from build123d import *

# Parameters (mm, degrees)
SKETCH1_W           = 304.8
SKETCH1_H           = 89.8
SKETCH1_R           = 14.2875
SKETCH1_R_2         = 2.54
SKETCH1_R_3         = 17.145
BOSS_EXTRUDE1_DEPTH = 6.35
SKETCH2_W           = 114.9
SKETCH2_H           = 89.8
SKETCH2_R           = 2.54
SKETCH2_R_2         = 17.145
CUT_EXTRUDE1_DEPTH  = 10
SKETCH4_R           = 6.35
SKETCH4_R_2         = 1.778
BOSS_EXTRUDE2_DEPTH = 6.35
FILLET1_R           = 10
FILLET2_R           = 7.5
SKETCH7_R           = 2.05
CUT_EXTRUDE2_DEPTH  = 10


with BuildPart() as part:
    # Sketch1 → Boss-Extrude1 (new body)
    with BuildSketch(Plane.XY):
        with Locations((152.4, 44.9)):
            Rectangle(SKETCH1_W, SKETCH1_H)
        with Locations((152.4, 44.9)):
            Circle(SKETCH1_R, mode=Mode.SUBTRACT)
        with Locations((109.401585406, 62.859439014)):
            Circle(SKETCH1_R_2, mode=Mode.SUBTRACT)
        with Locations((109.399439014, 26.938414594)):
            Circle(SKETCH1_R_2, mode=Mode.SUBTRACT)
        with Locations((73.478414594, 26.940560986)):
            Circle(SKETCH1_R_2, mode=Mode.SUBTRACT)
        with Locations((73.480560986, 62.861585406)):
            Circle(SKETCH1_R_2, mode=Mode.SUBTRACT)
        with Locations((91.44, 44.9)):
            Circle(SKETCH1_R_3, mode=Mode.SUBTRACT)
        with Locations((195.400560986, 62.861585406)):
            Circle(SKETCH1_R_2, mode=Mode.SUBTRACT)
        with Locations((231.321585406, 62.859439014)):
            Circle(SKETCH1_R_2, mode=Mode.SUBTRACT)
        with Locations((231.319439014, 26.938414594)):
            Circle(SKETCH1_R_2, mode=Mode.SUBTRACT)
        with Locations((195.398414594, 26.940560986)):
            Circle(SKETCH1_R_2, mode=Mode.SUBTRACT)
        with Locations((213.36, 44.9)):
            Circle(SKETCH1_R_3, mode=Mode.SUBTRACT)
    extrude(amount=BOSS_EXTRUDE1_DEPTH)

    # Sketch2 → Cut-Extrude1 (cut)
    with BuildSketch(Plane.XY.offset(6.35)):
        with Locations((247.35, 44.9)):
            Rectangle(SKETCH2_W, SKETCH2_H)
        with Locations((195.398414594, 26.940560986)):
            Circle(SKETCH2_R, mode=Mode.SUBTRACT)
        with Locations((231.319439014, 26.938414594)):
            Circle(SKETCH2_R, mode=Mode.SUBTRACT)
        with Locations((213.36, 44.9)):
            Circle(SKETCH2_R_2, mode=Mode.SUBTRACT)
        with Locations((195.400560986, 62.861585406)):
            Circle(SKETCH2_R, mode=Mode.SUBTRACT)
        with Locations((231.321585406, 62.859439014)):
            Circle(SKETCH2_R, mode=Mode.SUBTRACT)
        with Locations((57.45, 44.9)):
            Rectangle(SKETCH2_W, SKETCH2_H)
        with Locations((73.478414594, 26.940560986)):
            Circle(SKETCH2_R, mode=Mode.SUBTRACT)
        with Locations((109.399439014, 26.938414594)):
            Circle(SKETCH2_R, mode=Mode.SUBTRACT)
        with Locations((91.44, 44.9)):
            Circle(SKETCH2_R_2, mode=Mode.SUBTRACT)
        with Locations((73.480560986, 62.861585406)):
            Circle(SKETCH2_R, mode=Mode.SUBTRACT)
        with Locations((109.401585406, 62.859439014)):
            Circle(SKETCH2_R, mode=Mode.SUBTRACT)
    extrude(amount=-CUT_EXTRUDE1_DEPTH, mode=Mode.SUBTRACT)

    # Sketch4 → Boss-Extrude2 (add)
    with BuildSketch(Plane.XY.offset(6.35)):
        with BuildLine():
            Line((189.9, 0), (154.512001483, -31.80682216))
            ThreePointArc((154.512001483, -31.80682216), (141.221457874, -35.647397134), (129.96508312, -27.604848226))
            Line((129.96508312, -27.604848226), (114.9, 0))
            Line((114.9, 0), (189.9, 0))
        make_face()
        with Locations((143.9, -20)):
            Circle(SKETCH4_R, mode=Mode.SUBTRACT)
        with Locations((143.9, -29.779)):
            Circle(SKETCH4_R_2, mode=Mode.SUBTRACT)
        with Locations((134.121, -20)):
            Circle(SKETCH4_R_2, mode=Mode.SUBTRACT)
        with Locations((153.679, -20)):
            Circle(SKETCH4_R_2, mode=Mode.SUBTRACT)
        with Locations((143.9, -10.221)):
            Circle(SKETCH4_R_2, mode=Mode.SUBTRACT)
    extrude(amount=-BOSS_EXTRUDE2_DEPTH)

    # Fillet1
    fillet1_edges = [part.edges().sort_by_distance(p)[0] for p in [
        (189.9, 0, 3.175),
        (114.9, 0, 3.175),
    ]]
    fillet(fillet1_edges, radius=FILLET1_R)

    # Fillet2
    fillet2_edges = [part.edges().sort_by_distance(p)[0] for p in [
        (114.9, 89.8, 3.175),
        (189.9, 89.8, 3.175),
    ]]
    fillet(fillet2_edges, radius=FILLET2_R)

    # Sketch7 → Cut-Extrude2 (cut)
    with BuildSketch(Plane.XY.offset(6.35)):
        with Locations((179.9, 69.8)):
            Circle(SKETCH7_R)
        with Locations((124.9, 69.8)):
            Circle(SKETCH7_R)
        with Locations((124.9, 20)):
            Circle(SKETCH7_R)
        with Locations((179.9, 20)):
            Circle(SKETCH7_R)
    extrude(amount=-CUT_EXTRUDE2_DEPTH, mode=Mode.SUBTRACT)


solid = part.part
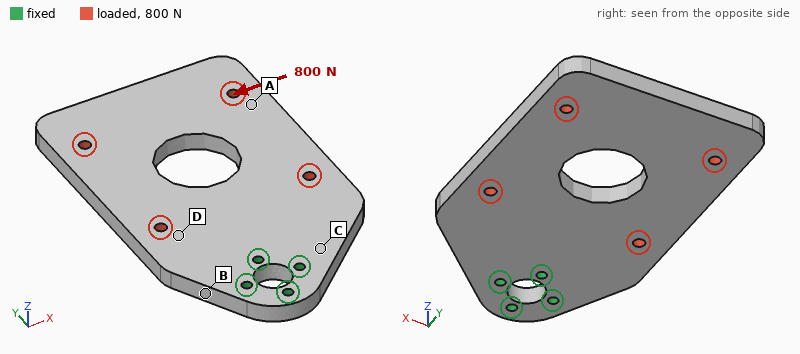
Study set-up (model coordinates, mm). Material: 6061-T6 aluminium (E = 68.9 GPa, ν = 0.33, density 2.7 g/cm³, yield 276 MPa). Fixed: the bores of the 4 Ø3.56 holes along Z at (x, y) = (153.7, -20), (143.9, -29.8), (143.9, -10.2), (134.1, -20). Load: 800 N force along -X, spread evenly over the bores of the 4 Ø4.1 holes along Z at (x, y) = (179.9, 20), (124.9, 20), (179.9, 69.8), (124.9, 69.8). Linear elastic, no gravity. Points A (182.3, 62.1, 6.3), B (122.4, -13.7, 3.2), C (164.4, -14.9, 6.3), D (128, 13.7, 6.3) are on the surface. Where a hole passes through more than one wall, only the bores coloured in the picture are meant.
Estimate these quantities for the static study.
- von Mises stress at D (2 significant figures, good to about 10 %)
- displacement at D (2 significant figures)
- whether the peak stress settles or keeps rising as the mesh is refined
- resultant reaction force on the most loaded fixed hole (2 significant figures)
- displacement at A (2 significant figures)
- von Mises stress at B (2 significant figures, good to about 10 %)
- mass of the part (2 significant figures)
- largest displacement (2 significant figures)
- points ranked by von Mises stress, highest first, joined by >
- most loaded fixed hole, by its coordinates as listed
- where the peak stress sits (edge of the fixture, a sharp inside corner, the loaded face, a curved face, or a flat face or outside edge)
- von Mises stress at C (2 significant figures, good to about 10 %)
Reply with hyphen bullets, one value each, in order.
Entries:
- 5.3 MPa
- 16 µm
- keeps rising
- 1.8 kN
- 46 µm
- 16 MPa
- 130 g
- 59 µm
- B > C > D > A
- (143.9, -10.2)
- edge of the fixture
- 11 MPa
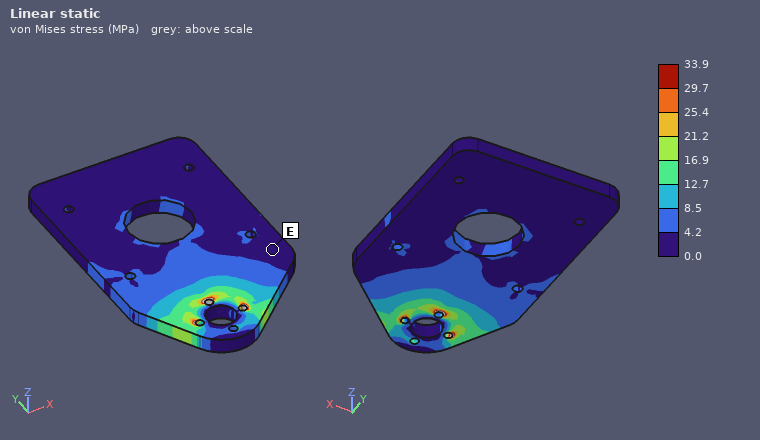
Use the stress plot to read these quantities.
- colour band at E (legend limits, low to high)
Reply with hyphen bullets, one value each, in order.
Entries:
- 0.0 to 4.2 MPa
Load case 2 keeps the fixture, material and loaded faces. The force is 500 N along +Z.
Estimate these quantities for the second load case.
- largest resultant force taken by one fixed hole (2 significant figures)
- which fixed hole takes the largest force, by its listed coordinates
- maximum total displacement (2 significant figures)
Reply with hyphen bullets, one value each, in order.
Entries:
- 1.5 kN
- (143.9, -10.2)
- 0.95 mm
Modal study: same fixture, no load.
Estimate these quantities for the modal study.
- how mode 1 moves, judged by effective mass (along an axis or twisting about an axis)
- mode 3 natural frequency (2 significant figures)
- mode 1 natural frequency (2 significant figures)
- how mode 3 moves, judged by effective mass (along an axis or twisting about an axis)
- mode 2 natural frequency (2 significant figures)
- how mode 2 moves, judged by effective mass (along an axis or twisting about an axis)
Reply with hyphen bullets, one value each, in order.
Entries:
- along Z
- 2100 Hz
- 450 Hz
- along X
- 1100 Hz
- twisting about Y
